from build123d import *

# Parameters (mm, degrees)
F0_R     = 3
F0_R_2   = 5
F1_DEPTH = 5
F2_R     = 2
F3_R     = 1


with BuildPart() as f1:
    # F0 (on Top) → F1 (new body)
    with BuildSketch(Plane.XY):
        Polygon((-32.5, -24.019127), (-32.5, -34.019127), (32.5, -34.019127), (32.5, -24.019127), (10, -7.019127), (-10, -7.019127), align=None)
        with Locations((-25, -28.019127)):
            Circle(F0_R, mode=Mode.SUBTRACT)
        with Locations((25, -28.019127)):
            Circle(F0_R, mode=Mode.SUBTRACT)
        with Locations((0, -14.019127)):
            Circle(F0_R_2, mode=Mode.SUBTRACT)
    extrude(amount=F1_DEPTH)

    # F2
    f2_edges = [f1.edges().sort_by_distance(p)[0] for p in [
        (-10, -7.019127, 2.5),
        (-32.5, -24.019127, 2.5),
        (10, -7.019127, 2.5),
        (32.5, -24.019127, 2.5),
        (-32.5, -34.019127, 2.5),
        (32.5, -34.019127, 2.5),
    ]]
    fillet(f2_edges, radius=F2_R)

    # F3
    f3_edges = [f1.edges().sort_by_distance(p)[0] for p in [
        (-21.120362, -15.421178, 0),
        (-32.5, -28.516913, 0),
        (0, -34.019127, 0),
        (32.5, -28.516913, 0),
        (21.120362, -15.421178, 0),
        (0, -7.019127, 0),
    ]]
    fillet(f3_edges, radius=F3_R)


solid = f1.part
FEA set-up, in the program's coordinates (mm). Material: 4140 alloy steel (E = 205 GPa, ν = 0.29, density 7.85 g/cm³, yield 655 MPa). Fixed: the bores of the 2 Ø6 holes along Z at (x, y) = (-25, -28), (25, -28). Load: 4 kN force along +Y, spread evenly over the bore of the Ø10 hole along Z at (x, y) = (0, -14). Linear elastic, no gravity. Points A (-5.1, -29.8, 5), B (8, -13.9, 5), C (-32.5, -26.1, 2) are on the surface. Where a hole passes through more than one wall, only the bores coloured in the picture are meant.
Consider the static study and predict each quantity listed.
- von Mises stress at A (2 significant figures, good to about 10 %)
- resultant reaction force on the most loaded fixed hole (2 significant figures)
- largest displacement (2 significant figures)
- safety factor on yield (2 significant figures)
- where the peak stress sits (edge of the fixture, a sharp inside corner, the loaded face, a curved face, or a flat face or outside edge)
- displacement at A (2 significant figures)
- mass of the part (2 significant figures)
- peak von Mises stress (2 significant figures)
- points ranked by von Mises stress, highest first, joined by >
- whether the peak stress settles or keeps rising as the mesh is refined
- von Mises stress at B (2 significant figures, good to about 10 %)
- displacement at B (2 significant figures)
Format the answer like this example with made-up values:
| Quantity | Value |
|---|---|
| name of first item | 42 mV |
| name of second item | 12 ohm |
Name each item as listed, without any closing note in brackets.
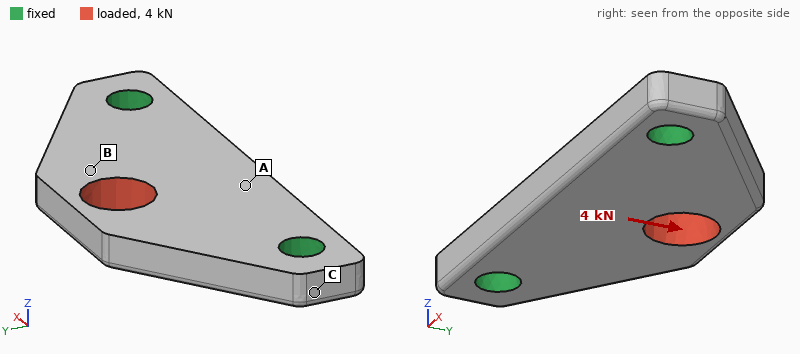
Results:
| Quantity | Value |
|---|---|
| von Mises stress at A | 22 MPa |
| resultant reaction force on the most loaded fixed hole | 2.3 kN |
| largest displacement | 11 µm |
| safety factor on yield | 3.9 |
| where the peak stress sits | a curved face |
| displacement at A | 7.8 µm |
| mass of the part | 48 g |
| peak von Mises stress | 170 MPa |
| points ranked by von Mises stress, highest first, joined by > | B > A > C |
| whether the peak stress settles or keeps rising as the mesh is refined | settles |
| von Mises stress at B | 43 MPa |
| displacement at B | 7.8 µm |
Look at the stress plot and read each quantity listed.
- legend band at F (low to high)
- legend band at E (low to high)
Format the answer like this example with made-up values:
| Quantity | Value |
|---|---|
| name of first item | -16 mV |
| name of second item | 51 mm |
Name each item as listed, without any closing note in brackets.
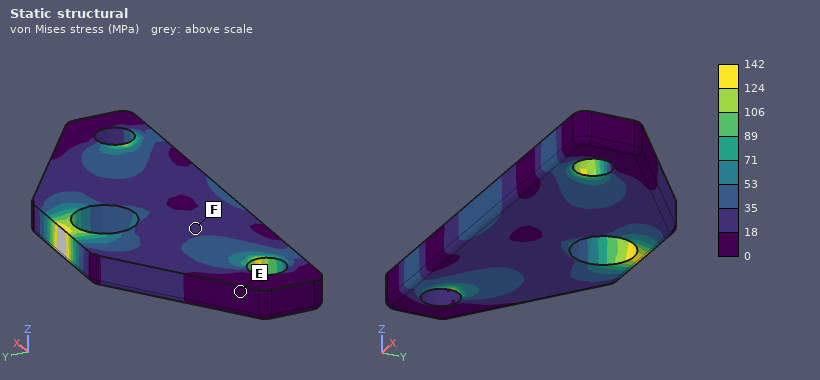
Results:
| Quantity | Value |
|---|---|
| legend band at F | 18 to 35 MPa |
| legend band at E | 0 to 18 MPa |
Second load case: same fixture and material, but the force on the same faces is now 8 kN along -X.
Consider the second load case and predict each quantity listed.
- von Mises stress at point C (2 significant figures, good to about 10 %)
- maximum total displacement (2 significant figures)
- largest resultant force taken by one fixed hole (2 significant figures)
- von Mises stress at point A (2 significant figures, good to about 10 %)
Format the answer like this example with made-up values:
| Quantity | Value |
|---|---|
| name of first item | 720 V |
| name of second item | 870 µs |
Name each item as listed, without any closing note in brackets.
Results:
| Quantity | Value |
|---|---|
| von Mises stress at point C | 20 MPa |
| maximum total displacement | 14 µm |
| largest resultant force taken by one fixed hole | 4.5 kN |
| von Mises stress at point A | 23 MPa |
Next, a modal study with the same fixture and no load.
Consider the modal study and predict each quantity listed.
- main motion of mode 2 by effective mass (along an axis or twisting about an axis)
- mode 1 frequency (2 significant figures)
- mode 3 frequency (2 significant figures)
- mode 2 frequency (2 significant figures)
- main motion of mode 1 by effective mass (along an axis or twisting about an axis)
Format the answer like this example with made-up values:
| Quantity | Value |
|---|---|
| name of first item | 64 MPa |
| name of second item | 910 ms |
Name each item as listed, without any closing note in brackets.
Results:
| Quantity | Value |
|---|---|
| main motion of mode 2 by effective mass | along Z |
| mode 1 frequency | 7300 Hz |
| mode 3 frequency | 17 kHz |
| mode 2 frequency | 13 kHz |
| main motion of mode 1 by effective mass | along Z |
